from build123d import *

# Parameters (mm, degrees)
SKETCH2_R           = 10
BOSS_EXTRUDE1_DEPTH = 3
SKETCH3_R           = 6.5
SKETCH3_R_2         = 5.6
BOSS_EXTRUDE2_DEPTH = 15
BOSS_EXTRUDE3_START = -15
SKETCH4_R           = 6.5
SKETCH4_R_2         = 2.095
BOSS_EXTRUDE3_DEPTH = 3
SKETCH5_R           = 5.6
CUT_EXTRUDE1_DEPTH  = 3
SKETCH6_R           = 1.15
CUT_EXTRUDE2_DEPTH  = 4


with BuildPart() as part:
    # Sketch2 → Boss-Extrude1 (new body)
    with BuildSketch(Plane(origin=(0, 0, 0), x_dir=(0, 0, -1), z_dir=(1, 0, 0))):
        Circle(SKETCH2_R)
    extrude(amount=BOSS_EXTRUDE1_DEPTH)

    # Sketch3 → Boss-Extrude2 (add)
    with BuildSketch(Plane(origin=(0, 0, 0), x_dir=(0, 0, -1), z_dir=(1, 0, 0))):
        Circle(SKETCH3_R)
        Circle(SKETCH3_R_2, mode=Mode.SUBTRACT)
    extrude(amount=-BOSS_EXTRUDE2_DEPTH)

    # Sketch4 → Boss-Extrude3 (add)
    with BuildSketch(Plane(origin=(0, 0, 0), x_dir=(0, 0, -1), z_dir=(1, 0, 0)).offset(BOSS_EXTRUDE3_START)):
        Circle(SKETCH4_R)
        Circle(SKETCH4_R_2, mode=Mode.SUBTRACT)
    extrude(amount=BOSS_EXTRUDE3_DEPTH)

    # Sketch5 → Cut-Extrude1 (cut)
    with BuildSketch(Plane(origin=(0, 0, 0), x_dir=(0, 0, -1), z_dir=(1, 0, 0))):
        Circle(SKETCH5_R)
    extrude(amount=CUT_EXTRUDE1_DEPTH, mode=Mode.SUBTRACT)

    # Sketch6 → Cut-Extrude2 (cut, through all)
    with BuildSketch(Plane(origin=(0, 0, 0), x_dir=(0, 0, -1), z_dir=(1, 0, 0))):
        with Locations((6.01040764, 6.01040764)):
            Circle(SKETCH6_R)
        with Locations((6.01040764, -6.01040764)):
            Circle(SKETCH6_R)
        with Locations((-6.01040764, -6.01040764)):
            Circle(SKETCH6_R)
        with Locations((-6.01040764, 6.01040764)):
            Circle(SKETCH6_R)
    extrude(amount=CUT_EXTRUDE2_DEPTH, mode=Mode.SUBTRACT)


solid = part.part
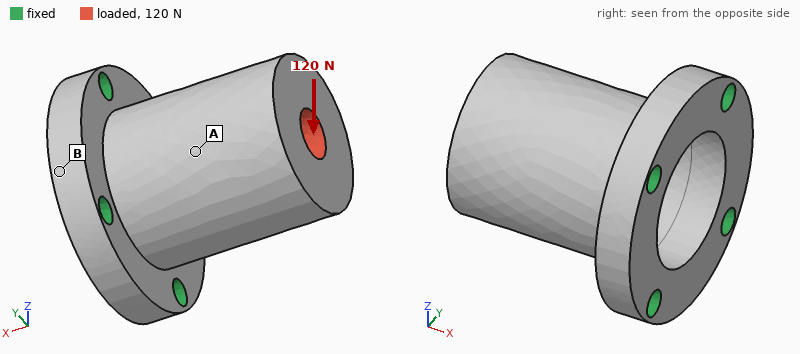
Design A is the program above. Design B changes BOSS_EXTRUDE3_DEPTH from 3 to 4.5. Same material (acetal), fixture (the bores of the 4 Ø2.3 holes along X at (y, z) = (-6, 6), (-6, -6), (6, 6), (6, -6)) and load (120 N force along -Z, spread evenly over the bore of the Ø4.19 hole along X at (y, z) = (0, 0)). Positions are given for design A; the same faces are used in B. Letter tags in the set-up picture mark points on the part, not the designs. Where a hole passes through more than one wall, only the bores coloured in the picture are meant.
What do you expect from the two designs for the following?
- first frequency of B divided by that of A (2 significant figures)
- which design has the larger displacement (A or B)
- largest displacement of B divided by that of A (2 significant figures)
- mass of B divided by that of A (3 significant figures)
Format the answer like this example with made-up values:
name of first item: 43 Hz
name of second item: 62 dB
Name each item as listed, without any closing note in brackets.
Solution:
first frequency of B divided by that of A: 0.93
which design has the larger displacement: A
largest displacement of B divided by that of A: 0.91
mass of B divided by that of A: 1.09
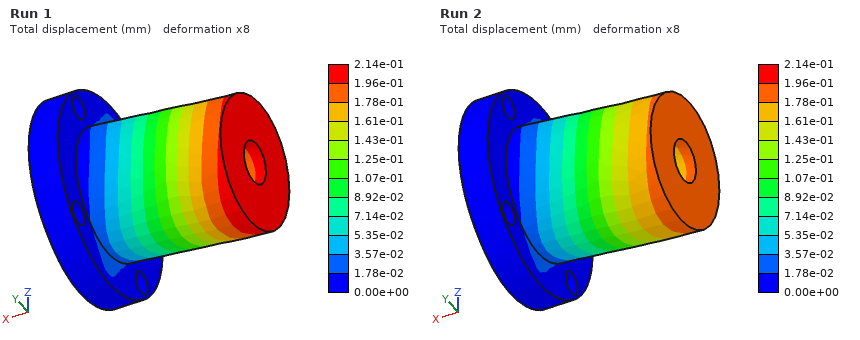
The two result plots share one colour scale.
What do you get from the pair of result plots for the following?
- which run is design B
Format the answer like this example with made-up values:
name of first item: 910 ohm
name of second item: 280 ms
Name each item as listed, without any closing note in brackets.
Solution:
which run is design B: Run 2
